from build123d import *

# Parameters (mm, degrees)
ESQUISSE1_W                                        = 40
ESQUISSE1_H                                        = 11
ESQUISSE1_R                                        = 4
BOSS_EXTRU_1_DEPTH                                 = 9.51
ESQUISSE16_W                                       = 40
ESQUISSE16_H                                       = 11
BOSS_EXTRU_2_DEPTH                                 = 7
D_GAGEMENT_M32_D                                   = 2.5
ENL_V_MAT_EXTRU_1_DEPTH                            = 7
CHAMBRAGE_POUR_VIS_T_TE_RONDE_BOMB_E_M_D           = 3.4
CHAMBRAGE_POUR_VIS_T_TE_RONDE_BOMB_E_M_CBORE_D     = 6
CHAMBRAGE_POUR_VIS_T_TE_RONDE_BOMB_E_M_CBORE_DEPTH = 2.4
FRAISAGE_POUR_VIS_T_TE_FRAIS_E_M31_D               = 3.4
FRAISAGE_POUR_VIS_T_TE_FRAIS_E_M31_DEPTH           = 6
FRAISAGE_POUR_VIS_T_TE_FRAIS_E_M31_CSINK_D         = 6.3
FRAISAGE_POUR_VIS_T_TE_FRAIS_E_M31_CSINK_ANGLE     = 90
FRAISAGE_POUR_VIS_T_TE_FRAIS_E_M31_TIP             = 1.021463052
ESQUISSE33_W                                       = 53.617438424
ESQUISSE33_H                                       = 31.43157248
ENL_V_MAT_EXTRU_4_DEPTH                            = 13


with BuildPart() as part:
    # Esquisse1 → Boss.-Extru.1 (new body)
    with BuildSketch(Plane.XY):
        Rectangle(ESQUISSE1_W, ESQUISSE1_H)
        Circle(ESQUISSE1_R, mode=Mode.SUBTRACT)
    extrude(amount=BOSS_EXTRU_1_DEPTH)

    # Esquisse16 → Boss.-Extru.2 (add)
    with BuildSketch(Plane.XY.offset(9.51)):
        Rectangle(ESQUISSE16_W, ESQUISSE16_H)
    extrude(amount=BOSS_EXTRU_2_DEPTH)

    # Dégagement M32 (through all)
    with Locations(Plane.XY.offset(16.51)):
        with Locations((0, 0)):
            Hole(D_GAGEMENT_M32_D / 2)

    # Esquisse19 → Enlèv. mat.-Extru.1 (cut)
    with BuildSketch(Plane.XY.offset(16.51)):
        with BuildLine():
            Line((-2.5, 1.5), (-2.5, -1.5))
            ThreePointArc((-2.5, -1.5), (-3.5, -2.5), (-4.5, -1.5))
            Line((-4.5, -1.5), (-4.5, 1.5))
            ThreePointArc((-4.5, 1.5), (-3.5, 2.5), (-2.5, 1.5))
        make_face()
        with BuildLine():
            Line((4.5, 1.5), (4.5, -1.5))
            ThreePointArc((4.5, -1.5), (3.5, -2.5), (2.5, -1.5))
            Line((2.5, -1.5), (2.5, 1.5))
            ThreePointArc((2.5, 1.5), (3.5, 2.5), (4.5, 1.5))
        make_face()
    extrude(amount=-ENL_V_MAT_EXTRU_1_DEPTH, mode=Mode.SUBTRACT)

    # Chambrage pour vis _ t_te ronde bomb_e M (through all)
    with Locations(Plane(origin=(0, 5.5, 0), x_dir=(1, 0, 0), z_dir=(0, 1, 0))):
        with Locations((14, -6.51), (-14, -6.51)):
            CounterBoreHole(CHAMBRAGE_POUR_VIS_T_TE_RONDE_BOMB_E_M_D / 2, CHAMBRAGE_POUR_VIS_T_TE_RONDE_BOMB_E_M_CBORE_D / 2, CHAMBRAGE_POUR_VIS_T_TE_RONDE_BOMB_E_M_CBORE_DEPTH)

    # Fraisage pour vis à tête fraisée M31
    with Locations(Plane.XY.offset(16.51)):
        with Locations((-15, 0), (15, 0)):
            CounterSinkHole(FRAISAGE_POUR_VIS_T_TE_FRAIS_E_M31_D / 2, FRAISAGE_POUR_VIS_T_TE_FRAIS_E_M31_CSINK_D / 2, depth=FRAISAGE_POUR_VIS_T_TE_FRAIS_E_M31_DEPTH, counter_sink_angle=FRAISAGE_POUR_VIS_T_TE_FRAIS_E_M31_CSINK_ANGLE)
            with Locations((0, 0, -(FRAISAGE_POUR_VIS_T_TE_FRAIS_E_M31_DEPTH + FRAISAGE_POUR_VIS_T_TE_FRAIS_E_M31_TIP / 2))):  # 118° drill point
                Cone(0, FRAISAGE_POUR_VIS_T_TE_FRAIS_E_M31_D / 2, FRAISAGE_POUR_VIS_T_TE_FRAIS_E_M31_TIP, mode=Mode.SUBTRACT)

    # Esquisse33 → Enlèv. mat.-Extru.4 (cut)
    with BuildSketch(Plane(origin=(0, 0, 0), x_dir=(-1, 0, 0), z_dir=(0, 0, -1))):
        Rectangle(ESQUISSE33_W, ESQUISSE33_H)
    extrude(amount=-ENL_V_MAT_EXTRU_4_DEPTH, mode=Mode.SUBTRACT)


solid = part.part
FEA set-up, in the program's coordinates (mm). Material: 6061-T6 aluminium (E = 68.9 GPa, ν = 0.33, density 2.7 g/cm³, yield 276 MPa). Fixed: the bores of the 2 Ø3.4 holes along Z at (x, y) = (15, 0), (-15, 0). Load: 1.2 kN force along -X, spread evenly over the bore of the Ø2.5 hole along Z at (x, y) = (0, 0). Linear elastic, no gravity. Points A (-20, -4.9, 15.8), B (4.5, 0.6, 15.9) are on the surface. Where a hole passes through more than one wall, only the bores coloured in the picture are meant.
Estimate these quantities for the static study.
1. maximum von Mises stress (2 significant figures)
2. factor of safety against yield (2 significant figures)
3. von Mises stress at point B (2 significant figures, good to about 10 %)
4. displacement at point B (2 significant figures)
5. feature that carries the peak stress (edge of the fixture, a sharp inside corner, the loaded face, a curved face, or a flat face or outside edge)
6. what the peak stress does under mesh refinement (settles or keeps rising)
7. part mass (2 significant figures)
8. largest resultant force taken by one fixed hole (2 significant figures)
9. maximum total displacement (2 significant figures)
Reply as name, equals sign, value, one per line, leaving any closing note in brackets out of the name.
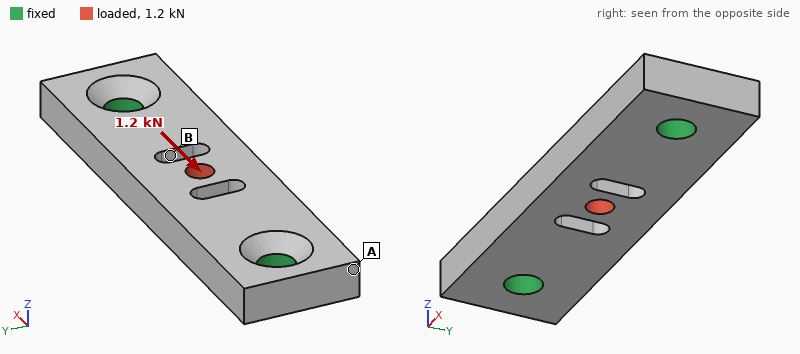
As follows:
maximum von Mises stress = 140 MPa
factor of safety against yield = 1.9
von Mises stress at point B = 32 MPa
displacement at point B = 2.3 µm
feature that carries the peak stress = a curved face
what the peak stress does under mesh refinement = settles
part mass = 3.7 g
largest resultant force taken by one fixed hole = 600 N
maximum total displacement = 11 µm
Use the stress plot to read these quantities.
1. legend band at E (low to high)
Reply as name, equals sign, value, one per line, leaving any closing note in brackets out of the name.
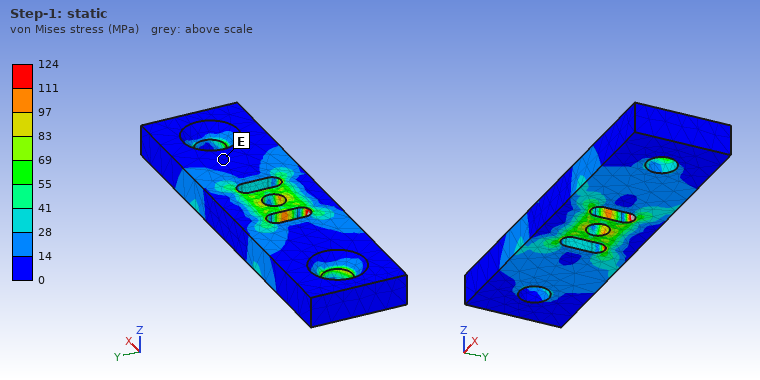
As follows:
legend band at E = 0 to 14 MPa
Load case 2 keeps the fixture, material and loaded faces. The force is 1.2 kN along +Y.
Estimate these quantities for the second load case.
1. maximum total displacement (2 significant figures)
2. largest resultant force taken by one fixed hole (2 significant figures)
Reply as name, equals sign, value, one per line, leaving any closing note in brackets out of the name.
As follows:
maximum total displacement = 29 µm
largest resultant force taken by one fixed hole = 600 N
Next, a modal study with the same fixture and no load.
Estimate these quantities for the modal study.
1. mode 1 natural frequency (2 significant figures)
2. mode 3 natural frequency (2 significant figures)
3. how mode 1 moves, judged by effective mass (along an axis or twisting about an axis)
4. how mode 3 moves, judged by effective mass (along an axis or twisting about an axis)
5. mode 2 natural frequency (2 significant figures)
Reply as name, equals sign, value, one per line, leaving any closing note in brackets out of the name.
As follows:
mode 1 natural frequency = 17 kHz
mode 3 natural frequency = 32 kHz
how mode 1 moves, judged by effective mass = along Z
how mode 3 moves, judged by effective mass = along Y
mode 2 natural frequency = 26 kHz
